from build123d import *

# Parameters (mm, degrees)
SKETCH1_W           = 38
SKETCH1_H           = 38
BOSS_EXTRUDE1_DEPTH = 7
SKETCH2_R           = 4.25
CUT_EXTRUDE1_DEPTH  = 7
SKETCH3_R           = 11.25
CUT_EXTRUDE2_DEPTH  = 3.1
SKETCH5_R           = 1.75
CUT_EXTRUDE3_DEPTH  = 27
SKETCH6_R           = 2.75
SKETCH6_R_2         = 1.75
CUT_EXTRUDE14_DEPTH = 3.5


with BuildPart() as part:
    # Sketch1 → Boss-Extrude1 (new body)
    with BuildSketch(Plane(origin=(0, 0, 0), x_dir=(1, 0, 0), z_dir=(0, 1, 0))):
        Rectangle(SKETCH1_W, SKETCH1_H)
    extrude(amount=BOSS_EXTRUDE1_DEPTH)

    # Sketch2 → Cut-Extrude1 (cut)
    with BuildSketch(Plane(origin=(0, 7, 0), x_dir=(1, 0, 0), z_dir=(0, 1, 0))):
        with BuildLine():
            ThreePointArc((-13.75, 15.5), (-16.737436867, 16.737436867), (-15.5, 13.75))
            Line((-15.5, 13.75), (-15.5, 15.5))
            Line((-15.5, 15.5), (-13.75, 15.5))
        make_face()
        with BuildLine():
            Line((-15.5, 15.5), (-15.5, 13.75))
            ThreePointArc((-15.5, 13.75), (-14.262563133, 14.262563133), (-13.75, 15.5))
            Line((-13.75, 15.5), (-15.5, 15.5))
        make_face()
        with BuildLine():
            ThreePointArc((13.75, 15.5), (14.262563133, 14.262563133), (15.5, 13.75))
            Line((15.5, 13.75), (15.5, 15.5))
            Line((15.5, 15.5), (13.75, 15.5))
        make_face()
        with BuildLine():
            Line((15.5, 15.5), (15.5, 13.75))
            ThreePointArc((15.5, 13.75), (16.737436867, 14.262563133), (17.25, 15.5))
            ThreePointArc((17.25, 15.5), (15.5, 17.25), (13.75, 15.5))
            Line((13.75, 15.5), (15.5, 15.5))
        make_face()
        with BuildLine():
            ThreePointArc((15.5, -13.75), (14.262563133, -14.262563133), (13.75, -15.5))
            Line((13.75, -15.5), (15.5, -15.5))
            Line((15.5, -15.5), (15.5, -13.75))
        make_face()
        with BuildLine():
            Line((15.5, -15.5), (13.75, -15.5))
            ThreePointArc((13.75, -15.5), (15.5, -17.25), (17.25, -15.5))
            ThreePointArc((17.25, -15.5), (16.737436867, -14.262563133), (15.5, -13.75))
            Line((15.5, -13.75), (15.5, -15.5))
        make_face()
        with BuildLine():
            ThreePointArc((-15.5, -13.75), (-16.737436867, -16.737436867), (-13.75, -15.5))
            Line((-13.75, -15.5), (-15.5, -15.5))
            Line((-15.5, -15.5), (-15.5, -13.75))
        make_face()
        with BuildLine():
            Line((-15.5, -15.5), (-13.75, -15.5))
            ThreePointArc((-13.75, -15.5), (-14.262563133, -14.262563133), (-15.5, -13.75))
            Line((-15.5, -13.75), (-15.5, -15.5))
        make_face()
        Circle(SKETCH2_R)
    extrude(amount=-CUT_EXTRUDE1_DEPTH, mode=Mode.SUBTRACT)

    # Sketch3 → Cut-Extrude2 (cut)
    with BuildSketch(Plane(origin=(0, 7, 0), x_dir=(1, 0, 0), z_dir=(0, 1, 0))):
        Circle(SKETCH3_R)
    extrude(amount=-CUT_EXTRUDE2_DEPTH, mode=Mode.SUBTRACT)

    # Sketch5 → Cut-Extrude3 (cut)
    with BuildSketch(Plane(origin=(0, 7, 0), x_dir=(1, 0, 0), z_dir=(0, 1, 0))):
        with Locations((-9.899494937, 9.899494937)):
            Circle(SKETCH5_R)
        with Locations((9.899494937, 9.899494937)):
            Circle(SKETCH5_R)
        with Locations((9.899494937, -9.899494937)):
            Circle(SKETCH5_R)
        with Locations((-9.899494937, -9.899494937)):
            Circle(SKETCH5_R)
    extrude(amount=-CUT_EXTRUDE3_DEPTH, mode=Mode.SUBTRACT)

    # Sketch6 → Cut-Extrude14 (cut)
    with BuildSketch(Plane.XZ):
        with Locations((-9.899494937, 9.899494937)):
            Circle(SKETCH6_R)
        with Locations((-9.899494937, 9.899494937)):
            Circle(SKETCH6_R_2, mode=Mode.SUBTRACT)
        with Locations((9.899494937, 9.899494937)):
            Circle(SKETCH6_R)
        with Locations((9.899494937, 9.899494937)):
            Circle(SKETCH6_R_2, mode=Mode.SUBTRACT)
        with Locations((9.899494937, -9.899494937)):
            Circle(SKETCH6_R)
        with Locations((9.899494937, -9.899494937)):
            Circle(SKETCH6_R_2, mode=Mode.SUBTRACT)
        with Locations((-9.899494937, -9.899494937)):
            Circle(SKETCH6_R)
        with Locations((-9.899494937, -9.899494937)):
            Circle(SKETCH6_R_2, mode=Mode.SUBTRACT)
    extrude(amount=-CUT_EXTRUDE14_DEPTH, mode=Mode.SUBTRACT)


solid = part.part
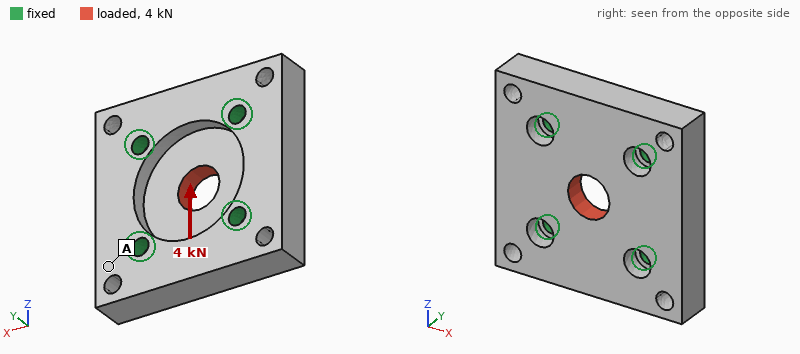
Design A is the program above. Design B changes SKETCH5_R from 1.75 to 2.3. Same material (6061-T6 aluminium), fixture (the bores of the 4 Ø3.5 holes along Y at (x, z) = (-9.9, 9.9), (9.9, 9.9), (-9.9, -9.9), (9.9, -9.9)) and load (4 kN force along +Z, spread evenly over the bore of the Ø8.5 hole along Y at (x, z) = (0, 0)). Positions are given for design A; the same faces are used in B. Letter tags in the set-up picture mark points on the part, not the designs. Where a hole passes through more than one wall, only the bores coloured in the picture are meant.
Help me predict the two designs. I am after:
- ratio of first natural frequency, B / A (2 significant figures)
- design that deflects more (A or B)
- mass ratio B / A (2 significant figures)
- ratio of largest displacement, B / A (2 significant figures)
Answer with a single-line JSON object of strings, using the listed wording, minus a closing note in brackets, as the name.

{"ratio of first natural frequency, B / A": "1.1", "design that deflects more": "A", "mass ratio B / A": "0.99", "ratio of largest displacement, B / A": "0.91"}
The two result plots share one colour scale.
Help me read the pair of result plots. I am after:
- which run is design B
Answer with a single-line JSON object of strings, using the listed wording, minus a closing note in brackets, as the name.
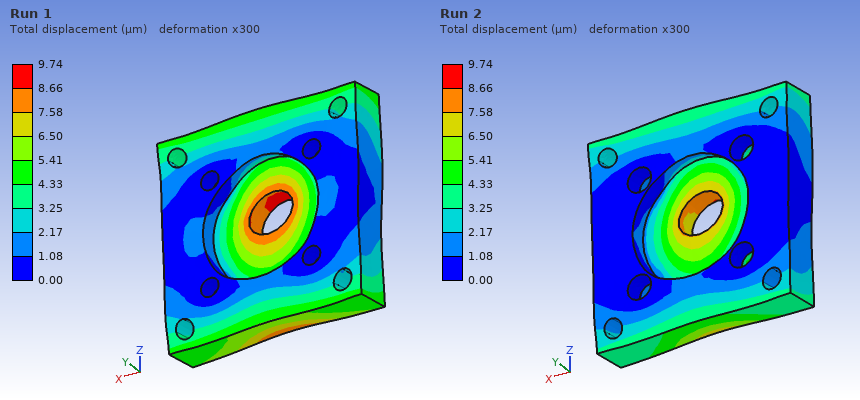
{"which run is design B": "Run 2"}
